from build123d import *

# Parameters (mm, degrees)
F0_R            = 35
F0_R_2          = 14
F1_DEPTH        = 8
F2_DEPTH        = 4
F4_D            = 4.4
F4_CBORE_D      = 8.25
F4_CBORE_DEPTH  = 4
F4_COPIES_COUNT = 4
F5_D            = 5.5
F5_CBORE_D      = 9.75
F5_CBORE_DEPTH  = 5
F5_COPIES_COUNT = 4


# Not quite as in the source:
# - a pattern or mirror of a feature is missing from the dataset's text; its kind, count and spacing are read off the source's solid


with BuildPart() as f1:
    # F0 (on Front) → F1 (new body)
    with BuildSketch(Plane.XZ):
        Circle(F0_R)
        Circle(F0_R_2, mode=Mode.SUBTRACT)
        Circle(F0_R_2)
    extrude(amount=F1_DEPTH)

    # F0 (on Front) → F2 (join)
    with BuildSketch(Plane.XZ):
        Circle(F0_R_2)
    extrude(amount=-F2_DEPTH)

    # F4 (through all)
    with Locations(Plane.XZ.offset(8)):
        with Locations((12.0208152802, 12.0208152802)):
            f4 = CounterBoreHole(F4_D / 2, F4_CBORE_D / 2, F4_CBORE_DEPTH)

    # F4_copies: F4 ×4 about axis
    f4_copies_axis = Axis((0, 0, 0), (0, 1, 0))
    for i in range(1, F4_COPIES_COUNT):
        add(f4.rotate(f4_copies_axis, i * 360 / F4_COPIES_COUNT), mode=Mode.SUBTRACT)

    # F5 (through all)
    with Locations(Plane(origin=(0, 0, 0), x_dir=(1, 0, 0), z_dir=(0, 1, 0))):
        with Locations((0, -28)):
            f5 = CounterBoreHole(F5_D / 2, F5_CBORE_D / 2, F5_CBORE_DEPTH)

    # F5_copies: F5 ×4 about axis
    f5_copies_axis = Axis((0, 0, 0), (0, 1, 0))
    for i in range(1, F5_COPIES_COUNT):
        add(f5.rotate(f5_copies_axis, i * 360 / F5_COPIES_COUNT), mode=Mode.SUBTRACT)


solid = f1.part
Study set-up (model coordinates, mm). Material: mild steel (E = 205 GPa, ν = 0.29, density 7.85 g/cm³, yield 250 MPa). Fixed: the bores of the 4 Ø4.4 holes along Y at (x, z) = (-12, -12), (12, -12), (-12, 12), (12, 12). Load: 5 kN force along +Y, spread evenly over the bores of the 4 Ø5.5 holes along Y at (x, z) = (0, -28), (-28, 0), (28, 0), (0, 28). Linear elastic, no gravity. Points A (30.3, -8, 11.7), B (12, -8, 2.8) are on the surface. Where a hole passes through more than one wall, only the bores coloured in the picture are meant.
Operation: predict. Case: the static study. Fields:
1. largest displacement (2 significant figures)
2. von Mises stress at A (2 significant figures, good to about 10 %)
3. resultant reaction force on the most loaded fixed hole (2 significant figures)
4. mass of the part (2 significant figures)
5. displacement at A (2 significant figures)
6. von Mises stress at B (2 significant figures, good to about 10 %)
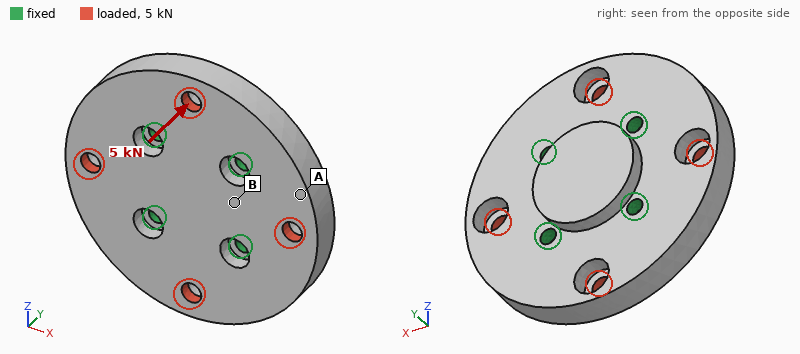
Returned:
12 µm
17 MPa
1.3 kN
240 g
7.5 µm
28 MPa
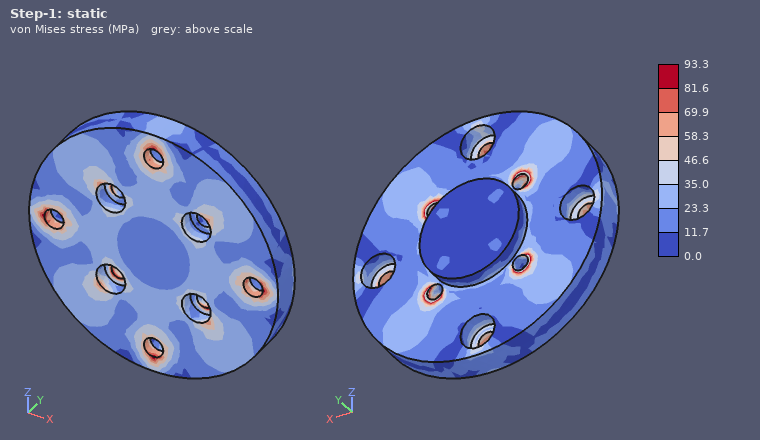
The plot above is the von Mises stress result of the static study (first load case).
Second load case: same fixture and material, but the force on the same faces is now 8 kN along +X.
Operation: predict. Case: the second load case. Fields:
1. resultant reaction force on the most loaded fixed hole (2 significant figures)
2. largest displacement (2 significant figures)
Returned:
2.2 kN
9.0 µm
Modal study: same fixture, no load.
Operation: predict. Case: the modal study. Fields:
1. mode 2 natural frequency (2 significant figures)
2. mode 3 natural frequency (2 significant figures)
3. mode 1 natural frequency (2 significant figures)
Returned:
11 kHz
11 kHz
11 kHz
